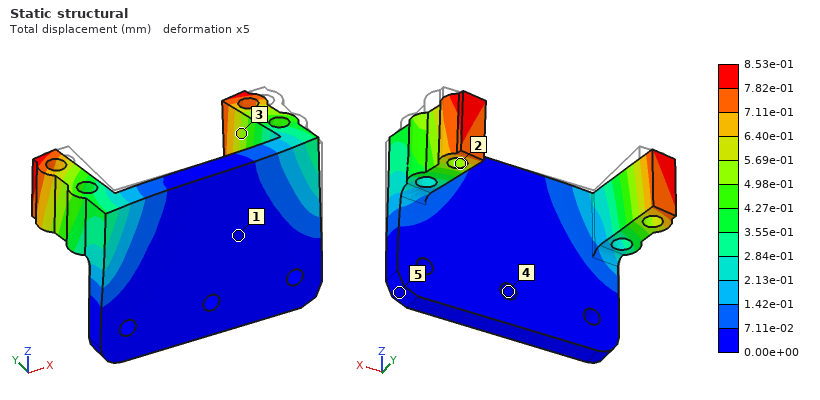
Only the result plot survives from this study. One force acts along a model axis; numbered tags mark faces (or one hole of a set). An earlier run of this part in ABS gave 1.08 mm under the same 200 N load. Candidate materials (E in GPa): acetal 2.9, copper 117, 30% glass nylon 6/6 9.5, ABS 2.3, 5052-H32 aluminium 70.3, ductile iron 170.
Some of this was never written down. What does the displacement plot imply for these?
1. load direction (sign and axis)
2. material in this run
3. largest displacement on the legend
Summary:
-X
acetal
8.53e-01 mm
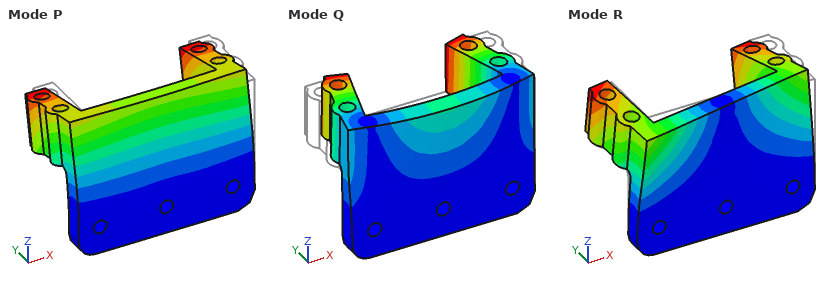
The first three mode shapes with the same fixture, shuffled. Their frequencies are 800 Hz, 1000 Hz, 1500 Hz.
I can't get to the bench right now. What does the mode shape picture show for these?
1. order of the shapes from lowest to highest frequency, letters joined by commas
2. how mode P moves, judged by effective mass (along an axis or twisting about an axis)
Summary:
P, R, Q
along Y
